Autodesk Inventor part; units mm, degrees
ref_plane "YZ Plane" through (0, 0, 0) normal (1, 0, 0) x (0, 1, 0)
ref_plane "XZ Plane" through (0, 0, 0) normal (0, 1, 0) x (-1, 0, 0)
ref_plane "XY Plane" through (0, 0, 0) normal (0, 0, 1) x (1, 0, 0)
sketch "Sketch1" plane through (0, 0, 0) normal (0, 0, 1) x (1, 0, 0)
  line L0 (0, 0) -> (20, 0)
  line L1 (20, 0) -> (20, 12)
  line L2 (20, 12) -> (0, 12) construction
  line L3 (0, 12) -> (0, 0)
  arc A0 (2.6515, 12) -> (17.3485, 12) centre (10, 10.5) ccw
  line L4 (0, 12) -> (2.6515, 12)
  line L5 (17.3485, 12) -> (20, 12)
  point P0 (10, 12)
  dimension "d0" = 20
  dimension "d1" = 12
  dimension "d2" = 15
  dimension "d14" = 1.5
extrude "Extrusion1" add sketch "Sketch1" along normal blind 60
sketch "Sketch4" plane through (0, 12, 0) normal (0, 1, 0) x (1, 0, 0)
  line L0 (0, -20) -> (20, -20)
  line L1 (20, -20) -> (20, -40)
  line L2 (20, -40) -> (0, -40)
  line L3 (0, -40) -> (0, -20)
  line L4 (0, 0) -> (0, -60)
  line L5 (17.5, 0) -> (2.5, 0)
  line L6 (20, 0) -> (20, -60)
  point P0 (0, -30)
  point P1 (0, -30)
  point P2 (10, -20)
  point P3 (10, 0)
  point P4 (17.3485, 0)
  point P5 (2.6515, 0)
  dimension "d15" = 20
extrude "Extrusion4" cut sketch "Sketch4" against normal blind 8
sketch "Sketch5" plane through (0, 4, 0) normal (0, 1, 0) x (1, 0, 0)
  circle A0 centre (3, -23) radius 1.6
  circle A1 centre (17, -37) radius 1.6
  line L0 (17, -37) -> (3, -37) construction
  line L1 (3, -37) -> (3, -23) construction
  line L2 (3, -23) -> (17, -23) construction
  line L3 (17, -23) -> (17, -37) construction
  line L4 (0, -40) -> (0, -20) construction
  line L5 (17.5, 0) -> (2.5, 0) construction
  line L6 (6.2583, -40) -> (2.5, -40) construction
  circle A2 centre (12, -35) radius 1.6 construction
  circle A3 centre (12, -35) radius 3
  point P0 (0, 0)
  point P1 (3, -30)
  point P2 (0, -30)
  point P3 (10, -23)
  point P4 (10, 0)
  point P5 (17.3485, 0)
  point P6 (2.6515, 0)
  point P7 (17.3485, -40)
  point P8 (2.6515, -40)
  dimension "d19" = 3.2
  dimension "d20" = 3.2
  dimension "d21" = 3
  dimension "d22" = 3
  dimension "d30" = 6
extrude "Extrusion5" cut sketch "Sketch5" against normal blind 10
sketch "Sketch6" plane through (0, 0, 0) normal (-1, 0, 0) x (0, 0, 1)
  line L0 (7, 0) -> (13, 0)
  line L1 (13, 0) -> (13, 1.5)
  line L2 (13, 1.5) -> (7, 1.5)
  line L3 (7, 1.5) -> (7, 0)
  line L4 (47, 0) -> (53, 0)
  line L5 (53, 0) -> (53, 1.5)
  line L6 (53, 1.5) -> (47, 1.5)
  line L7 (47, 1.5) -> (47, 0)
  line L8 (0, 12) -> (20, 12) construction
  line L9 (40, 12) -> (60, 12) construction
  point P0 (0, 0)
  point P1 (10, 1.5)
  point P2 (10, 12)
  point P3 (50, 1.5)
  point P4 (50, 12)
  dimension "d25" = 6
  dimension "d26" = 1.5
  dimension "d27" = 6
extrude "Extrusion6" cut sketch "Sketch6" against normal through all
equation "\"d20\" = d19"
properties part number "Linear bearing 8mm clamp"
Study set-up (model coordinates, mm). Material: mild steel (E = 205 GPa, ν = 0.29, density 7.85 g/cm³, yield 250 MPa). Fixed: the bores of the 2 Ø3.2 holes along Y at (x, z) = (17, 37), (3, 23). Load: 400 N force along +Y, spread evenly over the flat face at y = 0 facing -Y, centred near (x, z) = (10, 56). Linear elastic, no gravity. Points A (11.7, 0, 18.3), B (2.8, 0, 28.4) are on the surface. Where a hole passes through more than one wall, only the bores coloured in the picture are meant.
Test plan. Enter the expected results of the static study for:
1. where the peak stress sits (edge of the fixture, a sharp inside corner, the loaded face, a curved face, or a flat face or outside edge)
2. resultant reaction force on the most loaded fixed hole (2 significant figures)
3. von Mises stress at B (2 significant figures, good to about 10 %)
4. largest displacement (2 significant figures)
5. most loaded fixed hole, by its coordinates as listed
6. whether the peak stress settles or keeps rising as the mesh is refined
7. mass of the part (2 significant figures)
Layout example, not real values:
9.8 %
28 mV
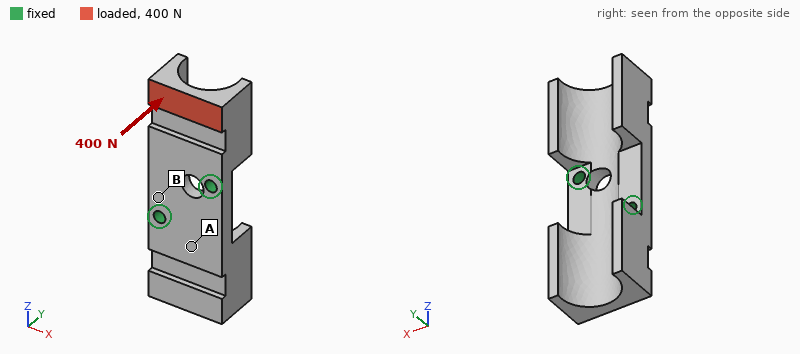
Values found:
edge of the fixture
460 N
56 MPa
90 µm
(17, 37)
keeps rising
48 g
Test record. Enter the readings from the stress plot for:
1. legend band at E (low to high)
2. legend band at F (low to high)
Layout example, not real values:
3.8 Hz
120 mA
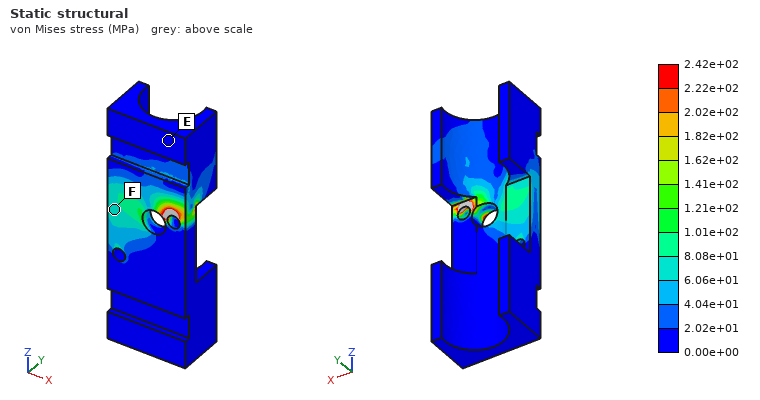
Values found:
0.00e+00 to 2.02e+01 MPa
6.06e+01 to 8.08e+01 MPa
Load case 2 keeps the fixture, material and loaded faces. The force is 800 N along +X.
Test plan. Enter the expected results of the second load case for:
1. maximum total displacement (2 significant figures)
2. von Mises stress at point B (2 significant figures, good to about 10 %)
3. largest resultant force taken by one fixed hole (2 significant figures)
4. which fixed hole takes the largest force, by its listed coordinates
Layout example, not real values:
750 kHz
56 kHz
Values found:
27 µm
23 MPa
1.3 kN
(17, 37)
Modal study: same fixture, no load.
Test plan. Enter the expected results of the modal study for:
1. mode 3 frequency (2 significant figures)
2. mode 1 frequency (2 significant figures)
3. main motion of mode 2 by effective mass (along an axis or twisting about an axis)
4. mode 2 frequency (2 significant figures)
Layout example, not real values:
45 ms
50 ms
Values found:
7700 Hz
3800 Hz
along Y
4000 Hz
